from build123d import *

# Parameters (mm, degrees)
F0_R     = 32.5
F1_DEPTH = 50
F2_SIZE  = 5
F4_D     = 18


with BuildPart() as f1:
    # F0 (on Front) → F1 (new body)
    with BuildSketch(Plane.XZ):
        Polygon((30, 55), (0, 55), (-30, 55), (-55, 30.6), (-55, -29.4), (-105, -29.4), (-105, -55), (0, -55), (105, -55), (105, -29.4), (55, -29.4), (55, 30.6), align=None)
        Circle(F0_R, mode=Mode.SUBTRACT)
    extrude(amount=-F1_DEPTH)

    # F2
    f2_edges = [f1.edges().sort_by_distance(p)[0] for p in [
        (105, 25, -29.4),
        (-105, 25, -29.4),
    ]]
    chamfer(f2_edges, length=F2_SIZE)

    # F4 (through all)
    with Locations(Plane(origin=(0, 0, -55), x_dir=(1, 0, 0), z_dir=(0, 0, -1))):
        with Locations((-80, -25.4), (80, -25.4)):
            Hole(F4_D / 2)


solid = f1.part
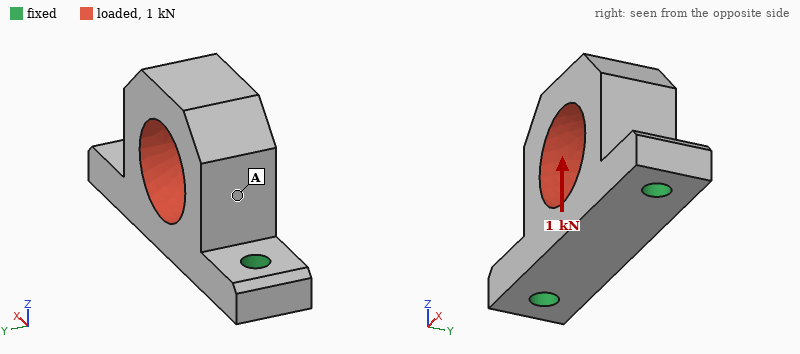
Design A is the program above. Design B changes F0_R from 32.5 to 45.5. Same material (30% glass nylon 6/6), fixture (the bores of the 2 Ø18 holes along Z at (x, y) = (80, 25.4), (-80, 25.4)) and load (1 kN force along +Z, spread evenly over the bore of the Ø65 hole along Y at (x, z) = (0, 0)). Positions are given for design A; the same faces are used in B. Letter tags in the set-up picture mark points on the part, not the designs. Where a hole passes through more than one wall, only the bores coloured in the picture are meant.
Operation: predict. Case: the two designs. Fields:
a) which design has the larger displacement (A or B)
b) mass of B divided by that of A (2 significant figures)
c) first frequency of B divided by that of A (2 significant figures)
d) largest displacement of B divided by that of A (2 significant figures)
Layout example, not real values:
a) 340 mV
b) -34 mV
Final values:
a) B
b) 0.70
c) 1.1
d) 1.5
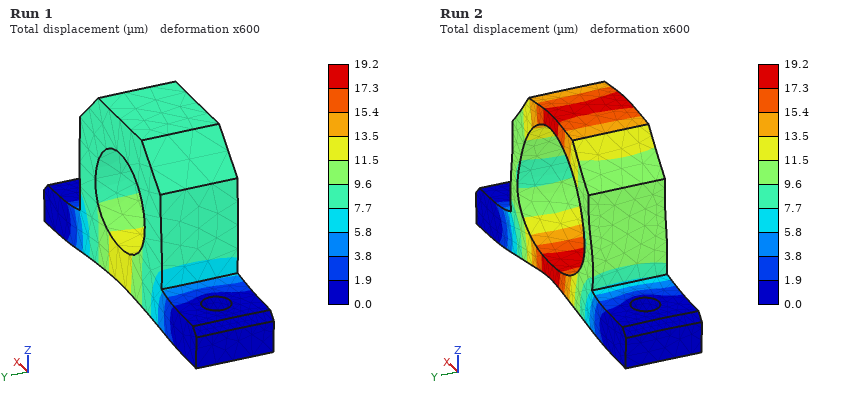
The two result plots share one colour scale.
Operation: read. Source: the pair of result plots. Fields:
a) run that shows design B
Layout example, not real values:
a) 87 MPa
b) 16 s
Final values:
a) Run 2
